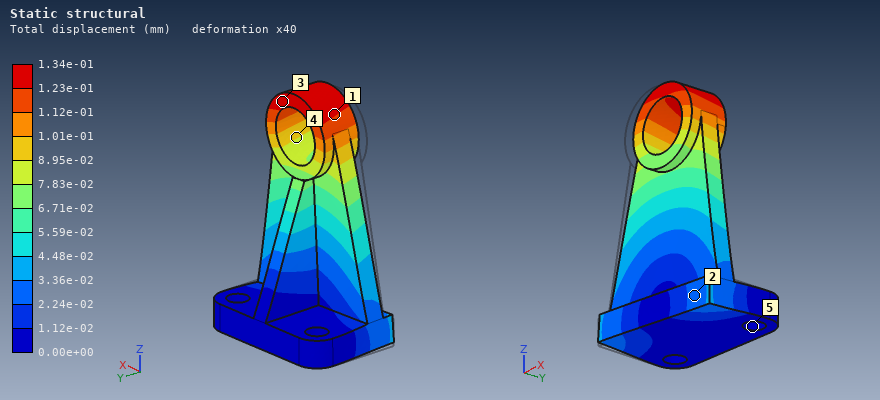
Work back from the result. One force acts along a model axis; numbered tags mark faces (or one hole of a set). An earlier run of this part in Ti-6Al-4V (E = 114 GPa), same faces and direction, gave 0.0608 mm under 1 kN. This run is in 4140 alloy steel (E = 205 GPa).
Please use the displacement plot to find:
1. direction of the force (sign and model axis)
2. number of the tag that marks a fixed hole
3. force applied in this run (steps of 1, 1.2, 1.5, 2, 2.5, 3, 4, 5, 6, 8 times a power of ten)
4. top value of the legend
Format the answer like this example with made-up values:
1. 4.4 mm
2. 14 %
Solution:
1. +X
2. 5
3. 4 kN
4. 1.34e-01 mm
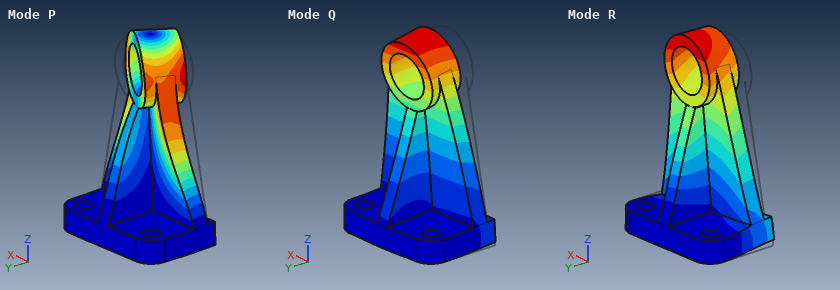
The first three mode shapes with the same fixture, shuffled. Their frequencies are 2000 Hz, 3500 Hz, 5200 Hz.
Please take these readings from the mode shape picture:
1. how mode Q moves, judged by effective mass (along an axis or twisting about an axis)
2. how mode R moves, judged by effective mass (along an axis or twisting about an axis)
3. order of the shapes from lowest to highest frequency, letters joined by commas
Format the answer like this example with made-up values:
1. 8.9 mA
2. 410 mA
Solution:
1. along Y
2. along X
3. Q, R, P
